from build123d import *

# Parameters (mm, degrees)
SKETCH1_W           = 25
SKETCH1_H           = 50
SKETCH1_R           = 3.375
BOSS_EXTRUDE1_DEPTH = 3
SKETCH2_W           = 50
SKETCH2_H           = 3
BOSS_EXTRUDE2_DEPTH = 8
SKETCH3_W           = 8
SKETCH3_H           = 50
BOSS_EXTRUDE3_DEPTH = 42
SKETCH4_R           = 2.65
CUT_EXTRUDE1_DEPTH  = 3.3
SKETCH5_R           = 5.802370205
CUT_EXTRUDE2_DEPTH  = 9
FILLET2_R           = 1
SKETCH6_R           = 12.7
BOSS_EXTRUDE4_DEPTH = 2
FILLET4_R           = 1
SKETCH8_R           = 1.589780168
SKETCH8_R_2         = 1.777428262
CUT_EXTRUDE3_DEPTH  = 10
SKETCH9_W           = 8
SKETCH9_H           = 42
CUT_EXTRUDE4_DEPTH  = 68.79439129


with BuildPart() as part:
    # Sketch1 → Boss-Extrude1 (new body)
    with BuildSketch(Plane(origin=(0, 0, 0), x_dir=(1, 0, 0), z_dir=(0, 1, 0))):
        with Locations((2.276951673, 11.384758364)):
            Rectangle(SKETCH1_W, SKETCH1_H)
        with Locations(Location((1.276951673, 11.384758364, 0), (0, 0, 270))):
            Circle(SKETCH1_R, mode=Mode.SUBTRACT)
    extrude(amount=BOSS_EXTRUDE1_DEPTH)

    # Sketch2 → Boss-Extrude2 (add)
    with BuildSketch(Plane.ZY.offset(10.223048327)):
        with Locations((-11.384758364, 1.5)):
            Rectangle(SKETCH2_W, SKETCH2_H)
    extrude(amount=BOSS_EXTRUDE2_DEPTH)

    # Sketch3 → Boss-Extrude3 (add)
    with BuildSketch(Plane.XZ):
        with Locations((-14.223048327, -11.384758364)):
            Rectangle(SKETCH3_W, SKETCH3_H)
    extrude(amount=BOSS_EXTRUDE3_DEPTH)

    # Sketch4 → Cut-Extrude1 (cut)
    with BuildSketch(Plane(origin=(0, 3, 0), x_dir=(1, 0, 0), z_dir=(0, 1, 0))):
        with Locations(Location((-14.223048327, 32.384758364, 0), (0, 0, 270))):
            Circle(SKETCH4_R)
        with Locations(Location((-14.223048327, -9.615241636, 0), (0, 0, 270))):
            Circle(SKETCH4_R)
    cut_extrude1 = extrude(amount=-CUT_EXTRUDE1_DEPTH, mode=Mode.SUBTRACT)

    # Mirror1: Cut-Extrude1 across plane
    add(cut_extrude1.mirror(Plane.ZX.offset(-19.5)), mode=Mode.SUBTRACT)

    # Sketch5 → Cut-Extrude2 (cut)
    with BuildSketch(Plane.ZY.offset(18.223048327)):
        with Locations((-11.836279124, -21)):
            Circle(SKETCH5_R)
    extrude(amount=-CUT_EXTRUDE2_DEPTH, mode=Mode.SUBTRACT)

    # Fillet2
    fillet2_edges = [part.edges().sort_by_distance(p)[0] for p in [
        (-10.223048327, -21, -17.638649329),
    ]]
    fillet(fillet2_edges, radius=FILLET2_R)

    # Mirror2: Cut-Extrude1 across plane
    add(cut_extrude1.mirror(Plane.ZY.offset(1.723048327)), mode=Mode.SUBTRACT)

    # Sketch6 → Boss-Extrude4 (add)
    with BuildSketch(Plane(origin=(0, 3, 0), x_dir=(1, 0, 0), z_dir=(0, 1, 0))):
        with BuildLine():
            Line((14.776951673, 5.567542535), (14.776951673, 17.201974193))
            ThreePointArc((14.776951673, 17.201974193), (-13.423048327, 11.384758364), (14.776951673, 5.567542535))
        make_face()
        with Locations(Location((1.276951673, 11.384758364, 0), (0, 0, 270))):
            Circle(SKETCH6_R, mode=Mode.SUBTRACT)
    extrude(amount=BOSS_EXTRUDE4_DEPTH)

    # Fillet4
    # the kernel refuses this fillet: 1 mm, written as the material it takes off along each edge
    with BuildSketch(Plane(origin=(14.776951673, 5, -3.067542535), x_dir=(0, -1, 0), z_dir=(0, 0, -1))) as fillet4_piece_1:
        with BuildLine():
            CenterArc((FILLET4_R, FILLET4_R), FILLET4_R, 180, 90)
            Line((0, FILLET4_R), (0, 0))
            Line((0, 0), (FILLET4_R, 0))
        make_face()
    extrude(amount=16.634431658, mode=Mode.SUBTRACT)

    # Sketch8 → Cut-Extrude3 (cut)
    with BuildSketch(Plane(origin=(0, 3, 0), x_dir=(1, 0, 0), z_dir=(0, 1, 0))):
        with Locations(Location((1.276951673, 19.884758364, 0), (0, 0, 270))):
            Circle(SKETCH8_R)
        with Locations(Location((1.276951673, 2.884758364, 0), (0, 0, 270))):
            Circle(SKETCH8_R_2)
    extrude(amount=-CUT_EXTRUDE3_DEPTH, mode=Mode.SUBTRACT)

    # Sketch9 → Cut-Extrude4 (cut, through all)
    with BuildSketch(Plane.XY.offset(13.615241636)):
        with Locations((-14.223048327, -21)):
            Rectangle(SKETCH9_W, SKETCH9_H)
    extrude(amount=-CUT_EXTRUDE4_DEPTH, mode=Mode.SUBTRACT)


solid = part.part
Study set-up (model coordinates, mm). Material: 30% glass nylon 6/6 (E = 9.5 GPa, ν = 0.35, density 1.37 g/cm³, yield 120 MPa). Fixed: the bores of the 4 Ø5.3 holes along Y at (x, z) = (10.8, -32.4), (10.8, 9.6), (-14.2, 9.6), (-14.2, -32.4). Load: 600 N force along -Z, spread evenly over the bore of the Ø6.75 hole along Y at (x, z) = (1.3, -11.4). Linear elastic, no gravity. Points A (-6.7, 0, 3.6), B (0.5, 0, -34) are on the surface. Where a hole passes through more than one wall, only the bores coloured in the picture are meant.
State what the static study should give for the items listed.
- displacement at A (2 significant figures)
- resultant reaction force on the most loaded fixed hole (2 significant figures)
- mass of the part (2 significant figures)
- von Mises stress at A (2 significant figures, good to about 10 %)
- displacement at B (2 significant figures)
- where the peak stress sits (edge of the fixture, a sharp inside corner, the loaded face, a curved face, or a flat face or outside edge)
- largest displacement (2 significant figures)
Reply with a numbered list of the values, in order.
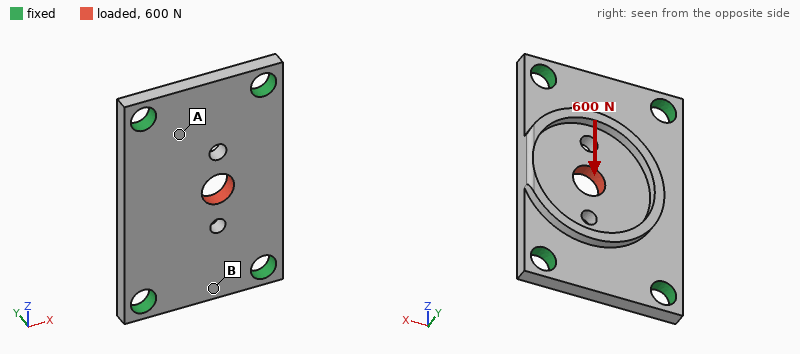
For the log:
1. 4.2 µm
2. 180 N
3. 6.6 g
4. 4.0 MPa
5. 4.4 µm
6. a curved face
7. 15 µm
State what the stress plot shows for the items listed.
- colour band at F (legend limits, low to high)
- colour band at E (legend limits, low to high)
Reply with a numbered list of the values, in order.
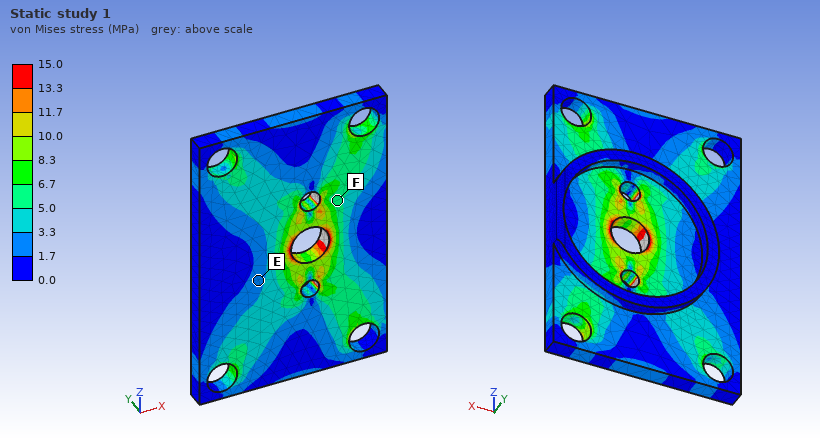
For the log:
1. 5.0 to 6.7 MPa
2. 1.7 to 3.3 MPa
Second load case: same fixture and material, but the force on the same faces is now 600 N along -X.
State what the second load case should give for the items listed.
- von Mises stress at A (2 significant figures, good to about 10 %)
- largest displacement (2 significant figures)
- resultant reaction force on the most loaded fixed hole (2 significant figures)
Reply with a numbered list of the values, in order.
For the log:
1. 6.1 MPa
2. 26 µm
3. 200 N
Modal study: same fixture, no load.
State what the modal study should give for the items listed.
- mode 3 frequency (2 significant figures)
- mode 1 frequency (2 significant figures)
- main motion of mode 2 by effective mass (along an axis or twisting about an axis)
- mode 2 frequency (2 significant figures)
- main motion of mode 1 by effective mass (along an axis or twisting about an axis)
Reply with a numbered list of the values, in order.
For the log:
1. 11 kHz
2. 5000 Hz
3. twisting about Z
4. 6800 Hz
5. along Y
